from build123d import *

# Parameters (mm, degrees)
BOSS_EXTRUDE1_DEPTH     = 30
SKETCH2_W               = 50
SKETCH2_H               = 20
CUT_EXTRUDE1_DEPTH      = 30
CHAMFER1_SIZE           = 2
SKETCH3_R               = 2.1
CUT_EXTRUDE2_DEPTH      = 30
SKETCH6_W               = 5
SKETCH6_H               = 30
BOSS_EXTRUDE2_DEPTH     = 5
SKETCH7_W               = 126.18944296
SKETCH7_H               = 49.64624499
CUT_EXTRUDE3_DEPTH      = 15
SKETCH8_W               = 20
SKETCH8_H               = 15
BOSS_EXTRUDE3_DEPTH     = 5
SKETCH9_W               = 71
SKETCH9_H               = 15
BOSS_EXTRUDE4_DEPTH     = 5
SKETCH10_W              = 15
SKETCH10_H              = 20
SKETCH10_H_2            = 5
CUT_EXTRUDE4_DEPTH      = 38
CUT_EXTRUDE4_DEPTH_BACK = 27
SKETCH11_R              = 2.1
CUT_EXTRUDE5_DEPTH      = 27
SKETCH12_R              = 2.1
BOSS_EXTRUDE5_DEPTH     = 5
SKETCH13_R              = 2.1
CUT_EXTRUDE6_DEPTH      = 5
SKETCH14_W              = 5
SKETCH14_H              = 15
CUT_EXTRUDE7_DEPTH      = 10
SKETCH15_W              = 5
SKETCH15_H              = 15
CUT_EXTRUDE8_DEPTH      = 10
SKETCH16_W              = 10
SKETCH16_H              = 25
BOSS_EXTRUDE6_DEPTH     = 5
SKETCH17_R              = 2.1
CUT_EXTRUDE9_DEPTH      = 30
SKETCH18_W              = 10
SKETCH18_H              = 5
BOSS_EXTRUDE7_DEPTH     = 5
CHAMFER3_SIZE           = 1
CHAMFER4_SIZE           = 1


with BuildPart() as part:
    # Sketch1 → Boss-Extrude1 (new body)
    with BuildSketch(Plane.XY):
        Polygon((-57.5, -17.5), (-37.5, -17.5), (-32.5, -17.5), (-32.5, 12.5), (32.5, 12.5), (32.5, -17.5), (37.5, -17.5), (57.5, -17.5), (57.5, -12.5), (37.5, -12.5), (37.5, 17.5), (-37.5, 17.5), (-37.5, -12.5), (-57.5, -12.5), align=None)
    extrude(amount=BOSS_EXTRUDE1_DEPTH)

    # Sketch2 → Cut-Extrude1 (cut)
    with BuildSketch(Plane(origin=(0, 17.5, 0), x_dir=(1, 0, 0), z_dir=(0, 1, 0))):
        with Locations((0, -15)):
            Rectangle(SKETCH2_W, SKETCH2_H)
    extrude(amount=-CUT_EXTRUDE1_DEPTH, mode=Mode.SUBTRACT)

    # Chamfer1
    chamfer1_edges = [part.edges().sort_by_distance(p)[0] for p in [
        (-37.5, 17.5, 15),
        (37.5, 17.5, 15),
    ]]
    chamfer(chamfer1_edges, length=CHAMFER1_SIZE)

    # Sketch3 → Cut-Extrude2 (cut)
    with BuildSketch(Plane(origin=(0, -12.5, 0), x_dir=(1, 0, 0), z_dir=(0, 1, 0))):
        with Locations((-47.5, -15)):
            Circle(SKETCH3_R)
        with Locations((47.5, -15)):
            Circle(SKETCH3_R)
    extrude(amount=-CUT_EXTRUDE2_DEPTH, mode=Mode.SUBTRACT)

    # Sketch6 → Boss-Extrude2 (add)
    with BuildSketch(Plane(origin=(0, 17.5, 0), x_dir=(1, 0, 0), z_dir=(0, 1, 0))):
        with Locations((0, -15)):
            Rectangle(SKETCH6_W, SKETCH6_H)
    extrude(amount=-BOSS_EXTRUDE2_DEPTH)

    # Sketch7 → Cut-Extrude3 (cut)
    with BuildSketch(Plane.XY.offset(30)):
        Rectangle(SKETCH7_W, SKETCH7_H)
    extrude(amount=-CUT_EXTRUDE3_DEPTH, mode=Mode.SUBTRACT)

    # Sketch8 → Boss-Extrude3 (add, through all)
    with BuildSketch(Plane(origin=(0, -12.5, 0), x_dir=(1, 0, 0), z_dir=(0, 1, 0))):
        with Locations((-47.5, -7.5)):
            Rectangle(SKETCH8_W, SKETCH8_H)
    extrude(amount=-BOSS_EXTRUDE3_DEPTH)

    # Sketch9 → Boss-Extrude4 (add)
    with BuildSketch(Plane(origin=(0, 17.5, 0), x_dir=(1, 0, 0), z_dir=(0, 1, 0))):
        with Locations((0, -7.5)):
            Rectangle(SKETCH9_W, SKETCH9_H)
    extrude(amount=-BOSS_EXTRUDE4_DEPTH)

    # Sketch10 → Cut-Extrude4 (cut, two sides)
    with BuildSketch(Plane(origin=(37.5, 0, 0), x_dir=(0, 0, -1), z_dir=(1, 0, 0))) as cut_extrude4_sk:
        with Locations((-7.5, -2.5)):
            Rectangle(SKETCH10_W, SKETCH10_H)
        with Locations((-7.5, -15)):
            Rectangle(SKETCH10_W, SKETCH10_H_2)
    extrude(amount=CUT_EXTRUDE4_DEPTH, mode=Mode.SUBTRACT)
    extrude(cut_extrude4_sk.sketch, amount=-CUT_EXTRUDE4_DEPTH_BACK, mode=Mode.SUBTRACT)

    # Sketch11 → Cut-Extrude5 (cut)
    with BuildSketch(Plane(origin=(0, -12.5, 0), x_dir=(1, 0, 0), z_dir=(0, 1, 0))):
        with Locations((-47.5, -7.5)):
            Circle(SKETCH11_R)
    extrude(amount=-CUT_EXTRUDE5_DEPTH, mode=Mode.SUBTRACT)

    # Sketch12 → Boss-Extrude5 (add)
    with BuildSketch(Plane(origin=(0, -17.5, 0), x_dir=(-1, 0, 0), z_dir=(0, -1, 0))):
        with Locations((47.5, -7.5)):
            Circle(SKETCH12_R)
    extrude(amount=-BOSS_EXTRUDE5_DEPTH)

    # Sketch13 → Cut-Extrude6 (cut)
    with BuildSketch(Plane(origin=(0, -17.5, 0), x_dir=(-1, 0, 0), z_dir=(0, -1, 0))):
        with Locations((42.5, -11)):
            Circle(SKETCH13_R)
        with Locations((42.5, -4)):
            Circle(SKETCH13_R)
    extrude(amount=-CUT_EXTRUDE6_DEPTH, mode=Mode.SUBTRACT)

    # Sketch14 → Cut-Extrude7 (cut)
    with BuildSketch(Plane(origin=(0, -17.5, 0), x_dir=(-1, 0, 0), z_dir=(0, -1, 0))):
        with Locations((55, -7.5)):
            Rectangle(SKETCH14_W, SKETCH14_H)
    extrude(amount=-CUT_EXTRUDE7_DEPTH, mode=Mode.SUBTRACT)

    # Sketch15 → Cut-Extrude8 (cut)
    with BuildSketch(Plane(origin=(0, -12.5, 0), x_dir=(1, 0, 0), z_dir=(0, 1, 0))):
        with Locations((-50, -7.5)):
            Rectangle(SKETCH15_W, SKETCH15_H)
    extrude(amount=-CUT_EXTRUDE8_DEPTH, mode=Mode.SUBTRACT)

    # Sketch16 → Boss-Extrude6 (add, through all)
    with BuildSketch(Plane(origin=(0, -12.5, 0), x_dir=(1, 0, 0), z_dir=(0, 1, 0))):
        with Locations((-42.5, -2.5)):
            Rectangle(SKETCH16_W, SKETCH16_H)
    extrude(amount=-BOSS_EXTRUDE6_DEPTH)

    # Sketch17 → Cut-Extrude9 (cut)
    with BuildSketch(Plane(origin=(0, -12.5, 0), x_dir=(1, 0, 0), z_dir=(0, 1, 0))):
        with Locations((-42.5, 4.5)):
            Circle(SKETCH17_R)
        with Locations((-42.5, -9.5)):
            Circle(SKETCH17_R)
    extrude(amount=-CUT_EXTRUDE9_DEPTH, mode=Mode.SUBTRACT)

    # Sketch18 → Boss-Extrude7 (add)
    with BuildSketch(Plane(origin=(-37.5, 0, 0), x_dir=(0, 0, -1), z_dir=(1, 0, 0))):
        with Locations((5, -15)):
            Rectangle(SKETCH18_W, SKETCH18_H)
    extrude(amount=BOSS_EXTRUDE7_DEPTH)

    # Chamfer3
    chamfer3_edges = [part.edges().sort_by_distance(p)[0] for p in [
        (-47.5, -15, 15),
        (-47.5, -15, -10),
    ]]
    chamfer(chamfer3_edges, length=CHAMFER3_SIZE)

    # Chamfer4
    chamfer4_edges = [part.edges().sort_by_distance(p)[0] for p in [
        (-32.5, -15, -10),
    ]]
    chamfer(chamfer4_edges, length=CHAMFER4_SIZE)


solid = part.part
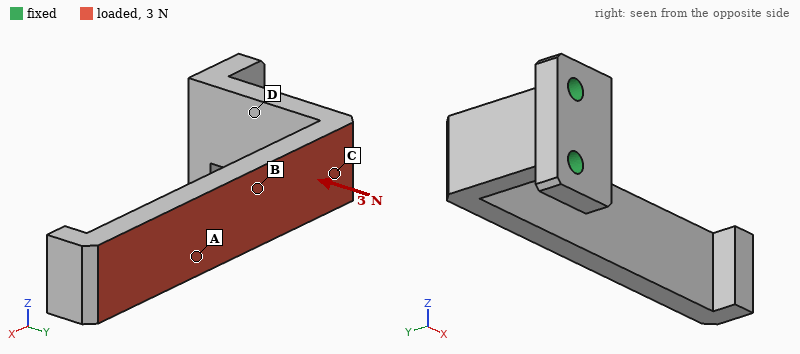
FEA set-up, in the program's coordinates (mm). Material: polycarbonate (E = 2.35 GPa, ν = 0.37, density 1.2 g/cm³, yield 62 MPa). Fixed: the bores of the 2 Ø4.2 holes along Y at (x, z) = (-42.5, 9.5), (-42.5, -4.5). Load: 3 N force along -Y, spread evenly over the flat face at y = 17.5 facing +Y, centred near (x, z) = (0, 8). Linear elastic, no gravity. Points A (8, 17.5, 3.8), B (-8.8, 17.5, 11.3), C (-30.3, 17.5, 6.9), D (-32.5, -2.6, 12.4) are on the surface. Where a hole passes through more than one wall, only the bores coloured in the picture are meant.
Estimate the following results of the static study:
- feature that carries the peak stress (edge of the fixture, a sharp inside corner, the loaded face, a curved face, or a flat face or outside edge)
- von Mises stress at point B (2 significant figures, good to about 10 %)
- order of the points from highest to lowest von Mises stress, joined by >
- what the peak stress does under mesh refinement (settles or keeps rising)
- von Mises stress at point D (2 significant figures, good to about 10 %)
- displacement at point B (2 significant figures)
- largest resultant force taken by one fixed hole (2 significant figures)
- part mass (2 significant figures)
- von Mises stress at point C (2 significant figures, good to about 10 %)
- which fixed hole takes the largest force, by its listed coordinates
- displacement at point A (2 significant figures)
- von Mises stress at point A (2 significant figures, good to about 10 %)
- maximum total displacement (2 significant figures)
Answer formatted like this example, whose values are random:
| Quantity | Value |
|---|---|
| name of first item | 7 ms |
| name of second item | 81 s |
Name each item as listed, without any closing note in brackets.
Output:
| Quantity | Value |
|---|---|
| feature that carries the peak stress | edge of the fixture |
| von Mises stress at point B | 0.67 MPa |
| order of the points from highest to lowest von Mises stress, joined by > | D > C > B > A |
| what the peak stress does under mesh refinement | keeps rising |
| von Mises stress at point D | 1.7 MPa |
| displacement at point B | 0.37 mm |
| largest resultant force taken by one fixed hole | 2.2 N |
| part mass | 11 g |
| von Mises stress at point C | 1.3 MPa |
| which fixed hole takes the largest force, by its listed coordinates | (-42.5, 9.5) |
| displacement at point A | 0.60 mm |
| von Mises stress at point A | 0.26 MPa |
| maximum total displacement | 1.0 mm |
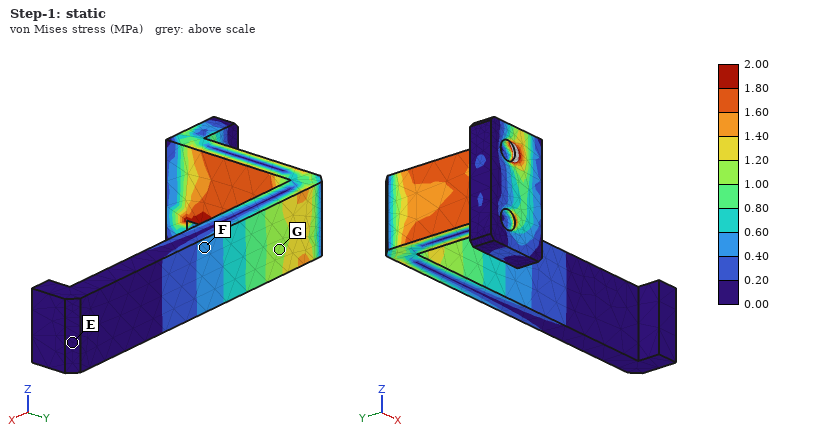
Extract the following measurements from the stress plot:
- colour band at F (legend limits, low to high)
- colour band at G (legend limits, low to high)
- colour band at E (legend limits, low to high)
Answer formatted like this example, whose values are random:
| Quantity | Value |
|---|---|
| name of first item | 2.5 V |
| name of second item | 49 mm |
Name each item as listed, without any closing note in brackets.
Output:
| Quantity | Value |
|---|---|
| colour band at F | 0.40 to 0.60 MPa |
| colour band at G | 1.00 to 1.20 MPa |
| colour band at E | 0.00 to 0.20 MPa |
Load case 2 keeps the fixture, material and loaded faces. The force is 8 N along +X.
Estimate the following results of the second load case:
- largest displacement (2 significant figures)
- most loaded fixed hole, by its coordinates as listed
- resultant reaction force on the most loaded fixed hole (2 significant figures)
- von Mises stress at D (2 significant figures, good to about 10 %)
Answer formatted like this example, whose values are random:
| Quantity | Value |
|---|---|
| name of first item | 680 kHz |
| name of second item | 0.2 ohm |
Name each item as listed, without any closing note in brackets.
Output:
| Quantity | Value |
|---|---|
| largest displacement | 1.1 mm |
| most loaded fixed hole, by its coordinates as listed | (-42.5, 9.5) |
| resultant reaction force on the most loaded fixed hole | 7.4 N |
| von Mises stress at D | 2.5 MPa |
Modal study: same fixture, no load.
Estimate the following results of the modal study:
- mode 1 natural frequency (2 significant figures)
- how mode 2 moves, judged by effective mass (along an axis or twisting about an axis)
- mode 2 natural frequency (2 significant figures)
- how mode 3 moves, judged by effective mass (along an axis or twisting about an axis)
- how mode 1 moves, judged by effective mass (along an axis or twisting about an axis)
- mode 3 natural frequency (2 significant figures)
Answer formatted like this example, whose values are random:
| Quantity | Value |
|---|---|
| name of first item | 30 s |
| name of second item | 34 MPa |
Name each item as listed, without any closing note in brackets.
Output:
| Quantity | Value |
|---|---|
| mode 1 natural frequency | 110 Hz |
| how mode 2 moves, judged by effective mass | along Z |
| mode 2 natural frequency | 170 Hz |
| how mode 3 moves, judged by effective mass | along X |
| how mode 1 moves, judged by effective mass | along Y |
| mode 3 natural frequency | 450 Hz |
